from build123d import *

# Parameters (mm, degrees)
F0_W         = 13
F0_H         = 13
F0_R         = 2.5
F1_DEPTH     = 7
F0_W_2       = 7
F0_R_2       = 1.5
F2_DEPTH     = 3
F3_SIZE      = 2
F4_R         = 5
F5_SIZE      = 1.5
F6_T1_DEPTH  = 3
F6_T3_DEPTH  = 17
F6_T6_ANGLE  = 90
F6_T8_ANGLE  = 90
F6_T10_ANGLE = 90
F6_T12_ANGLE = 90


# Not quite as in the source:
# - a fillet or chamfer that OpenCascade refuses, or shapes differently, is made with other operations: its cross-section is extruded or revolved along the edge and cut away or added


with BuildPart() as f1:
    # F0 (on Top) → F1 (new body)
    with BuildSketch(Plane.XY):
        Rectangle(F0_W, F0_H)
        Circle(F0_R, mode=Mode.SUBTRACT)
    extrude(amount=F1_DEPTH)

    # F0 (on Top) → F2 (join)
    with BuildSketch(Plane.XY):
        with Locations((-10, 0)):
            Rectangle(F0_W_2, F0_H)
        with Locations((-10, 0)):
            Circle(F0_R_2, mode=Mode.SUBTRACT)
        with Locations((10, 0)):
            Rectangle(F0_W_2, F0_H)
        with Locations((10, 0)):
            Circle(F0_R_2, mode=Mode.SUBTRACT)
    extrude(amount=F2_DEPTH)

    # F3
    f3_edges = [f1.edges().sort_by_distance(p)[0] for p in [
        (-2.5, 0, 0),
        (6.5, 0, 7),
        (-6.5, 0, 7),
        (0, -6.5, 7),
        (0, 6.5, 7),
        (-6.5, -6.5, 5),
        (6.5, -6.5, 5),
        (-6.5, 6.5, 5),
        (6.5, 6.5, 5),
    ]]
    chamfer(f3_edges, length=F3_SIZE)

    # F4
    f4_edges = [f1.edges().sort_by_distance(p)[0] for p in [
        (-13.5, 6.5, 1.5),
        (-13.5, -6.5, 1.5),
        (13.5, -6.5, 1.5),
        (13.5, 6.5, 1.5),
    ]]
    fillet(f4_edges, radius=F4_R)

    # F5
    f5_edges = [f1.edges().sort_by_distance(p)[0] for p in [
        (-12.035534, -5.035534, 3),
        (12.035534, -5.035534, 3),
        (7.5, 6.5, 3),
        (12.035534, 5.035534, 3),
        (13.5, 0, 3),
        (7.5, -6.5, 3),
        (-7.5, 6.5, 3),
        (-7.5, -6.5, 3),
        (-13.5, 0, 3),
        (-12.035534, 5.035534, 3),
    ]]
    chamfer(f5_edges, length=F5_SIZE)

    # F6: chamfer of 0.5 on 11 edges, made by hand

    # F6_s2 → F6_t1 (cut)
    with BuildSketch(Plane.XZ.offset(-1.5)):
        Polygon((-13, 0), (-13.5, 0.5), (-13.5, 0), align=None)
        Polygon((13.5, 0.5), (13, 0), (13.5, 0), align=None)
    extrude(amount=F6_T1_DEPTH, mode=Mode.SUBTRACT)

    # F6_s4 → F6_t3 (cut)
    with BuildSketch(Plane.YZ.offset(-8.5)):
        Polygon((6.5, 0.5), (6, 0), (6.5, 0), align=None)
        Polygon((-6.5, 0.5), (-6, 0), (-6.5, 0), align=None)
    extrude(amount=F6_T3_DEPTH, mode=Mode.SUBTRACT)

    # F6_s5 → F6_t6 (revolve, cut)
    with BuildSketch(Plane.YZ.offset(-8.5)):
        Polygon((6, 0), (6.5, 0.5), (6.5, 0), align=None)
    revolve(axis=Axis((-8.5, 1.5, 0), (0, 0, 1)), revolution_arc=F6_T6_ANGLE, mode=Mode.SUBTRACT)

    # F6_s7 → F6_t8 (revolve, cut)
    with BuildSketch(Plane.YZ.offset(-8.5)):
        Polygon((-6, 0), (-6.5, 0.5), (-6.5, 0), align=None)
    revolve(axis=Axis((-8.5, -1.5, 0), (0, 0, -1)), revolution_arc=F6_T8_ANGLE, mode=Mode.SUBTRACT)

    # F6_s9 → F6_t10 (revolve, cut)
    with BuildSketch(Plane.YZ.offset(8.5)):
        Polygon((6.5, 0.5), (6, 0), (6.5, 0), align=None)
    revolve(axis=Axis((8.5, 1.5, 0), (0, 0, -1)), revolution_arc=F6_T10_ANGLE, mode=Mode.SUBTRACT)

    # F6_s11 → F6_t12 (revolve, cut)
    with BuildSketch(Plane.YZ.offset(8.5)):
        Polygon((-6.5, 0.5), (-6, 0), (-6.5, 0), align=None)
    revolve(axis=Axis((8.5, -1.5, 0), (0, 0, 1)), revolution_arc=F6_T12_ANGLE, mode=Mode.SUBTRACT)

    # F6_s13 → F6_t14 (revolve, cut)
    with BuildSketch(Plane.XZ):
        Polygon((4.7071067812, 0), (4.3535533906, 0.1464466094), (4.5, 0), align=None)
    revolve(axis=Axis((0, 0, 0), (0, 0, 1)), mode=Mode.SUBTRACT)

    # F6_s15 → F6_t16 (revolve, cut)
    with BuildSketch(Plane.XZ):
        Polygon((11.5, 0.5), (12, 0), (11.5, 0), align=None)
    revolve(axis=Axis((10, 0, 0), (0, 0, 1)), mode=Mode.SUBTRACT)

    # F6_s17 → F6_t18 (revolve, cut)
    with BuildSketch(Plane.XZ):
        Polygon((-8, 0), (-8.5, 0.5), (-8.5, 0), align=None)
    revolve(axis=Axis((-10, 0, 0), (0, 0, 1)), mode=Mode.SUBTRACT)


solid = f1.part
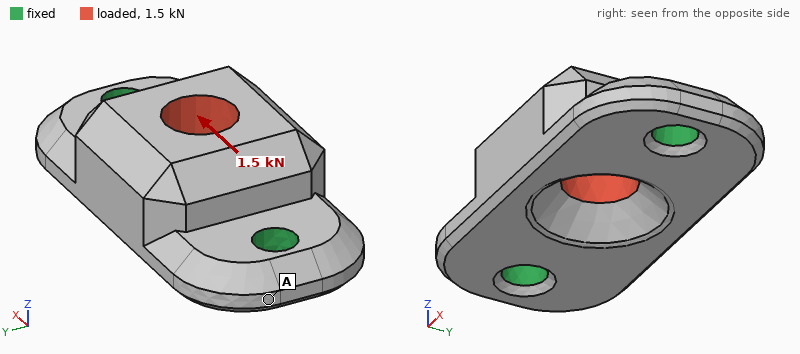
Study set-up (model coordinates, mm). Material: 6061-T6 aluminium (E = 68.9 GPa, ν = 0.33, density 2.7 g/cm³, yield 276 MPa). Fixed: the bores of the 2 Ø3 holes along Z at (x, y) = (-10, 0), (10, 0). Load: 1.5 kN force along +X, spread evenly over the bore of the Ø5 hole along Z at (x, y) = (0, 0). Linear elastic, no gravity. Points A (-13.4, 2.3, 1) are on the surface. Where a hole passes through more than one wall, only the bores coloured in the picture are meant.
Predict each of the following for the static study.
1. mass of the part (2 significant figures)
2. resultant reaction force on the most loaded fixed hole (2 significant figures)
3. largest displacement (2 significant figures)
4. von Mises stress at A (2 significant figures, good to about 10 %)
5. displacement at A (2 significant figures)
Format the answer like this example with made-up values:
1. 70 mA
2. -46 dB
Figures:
1. 3.4 g
2. 790 N
3. 6.5 µm
4. 12 MPa
5. 0.99 µm
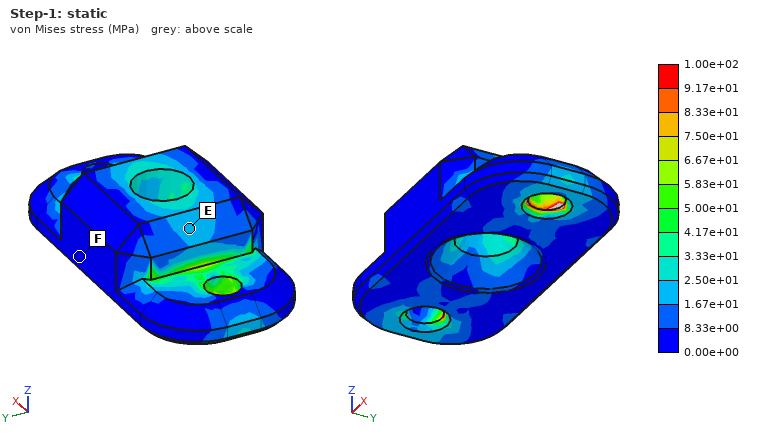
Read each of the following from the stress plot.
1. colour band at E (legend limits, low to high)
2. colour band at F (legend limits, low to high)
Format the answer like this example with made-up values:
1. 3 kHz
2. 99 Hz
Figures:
1. 1.67e+01 to 2.50e+01 MPa
2. 0.00e+00 to 8.33e+00 MPa
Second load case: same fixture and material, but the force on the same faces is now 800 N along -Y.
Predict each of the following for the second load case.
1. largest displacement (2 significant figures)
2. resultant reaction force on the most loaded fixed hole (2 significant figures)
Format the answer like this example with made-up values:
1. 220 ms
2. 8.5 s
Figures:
1. 17 µm
2. 400 N
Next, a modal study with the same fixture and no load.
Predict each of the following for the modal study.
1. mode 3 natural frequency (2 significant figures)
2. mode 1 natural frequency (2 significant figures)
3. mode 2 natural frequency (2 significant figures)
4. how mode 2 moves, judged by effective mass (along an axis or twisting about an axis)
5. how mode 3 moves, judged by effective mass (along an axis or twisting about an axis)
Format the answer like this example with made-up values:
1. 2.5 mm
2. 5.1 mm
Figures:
1. 53 kHz
2. 24 kHz
3. 34 kHz
4. along Z
5. along Y
